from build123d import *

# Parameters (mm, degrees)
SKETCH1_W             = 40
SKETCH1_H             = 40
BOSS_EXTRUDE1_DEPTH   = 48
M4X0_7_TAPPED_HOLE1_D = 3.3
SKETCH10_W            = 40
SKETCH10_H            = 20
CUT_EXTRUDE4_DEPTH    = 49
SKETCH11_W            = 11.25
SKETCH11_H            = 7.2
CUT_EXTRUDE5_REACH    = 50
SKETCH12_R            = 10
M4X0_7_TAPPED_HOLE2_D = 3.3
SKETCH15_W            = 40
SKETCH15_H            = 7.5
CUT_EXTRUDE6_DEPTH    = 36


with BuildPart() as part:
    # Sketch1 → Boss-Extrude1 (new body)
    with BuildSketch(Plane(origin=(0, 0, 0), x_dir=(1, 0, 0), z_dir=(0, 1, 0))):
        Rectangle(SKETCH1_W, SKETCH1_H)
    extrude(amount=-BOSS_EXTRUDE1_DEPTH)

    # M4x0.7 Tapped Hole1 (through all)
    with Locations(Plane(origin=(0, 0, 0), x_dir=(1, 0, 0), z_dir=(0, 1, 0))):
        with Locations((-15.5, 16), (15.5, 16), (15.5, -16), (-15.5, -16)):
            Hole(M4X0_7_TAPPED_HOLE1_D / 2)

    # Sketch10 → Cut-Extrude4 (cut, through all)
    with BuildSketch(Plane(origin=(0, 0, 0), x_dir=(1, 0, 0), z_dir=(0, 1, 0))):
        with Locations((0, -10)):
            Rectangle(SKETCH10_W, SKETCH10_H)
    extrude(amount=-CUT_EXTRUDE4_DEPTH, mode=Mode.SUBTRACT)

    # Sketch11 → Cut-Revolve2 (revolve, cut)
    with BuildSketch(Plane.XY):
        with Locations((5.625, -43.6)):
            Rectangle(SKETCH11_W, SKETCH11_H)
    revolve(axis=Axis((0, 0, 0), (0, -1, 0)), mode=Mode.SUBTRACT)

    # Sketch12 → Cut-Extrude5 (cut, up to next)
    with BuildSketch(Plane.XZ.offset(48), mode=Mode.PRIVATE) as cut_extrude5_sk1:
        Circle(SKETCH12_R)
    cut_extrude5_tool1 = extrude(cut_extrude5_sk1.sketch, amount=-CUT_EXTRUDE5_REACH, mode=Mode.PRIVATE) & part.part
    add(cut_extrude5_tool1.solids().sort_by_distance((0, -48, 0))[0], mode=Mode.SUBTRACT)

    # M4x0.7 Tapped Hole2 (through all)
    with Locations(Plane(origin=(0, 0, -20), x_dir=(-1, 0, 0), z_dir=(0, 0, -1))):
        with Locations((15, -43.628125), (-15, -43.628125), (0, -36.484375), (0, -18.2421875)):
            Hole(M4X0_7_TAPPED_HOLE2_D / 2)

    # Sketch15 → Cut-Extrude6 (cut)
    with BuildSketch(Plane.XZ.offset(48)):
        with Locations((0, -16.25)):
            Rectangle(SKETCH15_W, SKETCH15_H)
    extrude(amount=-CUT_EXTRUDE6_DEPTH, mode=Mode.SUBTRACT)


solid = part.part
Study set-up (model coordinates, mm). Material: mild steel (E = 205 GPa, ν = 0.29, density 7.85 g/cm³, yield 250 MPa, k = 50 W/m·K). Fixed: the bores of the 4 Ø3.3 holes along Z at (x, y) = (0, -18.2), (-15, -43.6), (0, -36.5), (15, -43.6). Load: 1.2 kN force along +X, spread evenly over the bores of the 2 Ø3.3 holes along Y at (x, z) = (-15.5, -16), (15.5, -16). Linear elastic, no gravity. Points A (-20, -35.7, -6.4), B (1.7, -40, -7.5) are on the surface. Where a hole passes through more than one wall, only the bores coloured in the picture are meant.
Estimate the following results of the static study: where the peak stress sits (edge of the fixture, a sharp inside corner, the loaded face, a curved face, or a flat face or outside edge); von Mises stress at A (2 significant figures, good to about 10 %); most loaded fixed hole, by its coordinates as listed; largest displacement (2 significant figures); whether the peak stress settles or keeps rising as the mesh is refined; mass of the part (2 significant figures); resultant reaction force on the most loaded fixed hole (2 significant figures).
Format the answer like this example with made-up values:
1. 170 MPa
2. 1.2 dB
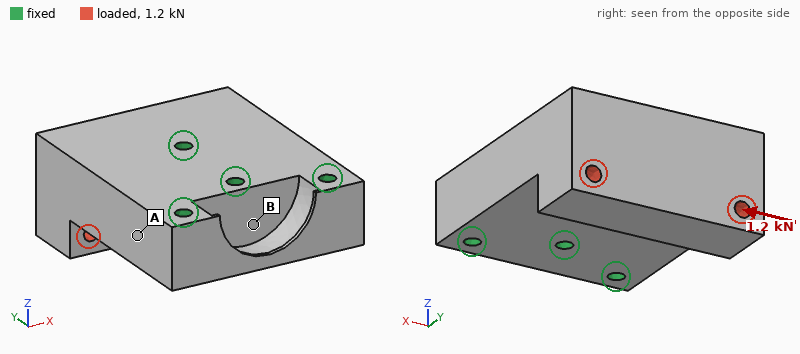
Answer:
1. edge of the fixture
2. 5.2 MPa
3. (0, -18.2)
4. 3.5 µm
5. keeps rising
6. 200 g
7. 1.4 kN
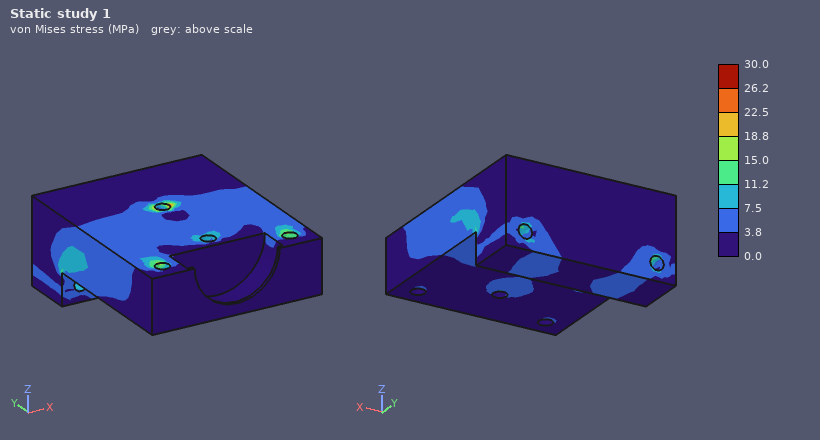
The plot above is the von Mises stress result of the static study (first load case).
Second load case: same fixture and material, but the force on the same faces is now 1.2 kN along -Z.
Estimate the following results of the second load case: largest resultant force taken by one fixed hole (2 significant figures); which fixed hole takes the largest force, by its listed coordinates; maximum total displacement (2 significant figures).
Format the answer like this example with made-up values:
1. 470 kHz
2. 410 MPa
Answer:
1. 1.4 kN
2. (0, -18.2)
3. 3.9 µm
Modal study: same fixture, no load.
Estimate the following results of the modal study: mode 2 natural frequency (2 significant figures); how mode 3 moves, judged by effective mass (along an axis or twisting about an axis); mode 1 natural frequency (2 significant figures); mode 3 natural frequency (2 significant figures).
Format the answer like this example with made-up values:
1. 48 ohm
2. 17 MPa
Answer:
1. 13 kHz
2. along X
3. 12 kHz
4. 19 kHz
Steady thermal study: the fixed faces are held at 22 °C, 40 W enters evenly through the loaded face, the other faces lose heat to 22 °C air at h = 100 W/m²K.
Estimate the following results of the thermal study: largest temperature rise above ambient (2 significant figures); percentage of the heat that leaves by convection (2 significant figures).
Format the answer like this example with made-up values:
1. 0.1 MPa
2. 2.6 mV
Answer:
1. 45 K
2. 21 %
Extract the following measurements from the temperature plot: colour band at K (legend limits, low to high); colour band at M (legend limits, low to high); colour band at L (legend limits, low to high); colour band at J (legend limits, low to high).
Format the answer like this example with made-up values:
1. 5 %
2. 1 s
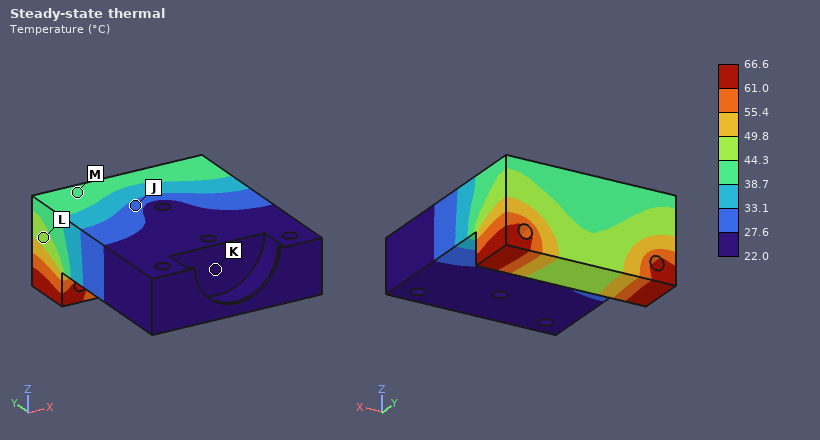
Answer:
1. 22.0 to 27.6 °C
2. 38.7 to 44.3 °C
3. 44.3 to 49.8 °C
4. 27.6 to 33.1 °C
